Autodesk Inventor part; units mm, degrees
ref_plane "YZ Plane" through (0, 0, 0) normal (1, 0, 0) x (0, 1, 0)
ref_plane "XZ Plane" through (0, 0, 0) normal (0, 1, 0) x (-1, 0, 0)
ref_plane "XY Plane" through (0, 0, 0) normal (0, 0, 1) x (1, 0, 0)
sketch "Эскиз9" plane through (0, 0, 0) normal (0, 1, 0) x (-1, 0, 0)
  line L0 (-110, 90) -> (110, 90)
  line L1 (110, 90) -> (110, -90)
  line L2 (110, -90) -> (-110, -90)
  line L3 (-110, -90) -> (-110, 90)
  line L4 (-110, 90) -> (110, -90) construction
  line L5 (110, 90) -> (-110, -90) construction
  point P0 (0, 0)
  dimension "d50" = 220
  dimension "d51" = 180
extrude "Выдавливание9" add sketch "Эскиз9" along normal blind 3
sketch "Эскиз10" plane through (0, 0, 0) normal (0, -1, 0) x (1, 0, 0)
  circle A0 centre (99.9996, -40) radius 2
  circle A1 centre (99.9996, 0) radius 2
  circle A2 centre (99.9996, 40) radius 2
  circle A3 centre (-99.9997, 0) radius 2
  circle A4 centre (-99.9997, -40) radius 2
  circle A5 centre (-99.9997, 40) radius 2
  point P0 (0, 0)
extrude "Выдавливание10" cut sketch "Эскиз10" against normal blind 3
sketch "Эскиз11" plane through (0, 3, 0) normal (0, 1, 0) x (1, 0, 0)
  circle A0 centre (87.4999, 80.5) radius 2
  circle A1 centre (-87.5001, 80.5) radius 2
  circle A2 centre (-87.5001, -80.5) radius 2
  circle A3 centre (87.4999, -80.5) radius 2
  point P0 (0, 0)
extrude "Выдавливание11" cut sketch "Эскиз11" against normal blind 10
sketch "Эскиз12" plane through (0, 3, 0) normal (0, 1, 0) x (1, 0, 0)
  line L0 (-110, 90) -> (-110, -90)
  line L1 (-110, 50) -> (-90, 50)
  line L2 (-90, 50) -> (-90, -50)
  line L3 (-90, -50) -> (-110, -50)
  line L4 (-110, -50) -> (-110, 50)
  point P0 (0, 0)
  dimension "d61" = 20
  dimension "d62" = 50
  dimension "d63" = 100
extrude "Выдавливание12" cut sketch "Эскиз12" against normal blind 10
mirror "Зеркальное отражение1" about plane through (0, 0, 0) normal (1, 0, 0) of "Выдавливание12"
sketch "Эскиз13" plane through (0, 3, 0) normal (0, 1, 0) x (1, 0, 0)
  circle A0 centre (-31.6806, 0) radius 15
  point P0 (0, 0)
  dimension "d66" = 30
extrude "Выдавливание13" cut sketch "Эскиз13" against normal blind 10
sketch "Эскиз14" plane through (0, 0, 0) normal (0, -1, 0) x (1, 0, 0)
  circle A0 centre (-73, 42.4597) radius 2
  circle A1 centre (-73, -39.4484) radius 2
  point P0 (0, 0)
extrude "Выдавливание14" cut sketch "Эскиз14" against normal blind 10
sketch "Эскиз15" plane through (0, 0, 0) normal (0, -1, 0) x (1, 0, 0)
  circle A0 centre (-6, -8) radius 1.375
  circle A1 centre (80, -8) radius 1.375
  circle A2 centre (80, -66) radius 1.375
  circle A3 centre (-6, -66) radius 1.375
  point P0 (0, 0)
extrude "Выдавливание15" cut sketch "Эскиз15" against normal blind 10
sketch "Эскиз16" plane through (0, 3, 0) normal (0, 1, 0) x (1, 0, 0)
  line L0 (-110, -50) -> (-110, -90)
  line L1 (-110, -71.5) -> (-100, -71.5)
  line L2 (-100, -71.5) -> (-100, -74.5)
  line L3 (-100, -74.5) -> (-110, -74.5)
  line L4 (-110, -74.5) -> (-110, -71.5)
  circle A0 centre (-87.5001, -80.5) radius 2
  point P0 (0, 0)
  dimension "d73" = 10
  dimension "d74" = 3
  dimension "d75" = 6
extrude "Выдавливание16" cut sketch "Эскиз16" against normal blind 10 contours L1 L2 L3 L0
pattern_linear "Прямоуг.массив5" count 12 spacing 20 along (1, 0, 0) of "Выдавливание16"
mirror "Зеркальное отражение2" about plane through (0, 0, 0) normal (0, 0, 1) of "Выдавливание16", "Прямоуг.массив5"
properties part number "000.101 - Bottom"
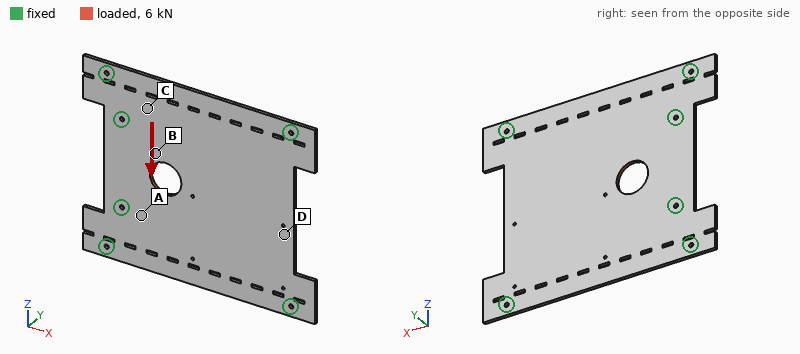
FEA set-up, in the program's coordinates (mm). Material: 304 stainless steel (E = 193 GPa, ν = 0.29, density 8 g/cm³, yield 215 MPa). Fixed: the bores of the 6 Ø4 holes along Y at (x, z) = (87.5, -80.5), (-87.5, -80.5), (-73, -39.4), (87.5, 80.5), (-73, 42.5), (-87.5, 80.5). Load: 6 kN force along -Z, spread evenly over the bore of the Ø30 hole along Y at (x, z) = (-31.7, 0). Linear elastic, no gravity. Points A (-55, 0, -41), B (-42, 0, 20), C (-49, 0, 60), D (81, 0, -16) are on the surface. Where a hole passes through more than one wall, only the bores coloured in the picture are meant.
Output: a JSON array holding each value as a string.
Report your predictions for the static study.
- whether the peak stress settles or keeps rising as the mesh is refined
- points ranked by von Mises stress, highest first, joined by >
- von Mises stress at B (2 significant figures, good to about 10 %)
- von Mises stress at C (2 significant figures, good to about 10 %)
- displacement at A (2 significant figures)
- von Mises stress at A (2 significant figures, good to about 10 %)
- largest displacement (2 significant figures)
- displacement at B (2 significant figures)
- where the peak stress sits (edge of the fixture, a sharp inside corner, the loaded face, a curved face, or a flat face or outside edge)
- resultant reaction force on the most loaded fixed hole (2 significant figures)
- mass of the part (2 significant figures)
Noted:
["keeps rising", "B > A > C > D", "21 MPa", "12 MPa", "3.8 µm", "16 MPa", "9.7 µm", "6.5 µm", "edge of the fixture", "1.9 kN", "820 g"]
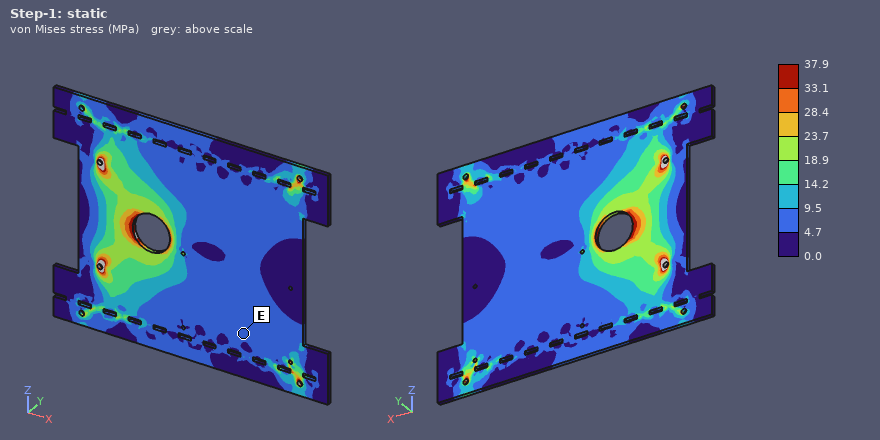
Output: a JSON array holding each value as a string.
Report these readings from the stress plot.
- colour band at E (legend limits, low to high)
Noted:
["4.7 to 9.5 MPa"]
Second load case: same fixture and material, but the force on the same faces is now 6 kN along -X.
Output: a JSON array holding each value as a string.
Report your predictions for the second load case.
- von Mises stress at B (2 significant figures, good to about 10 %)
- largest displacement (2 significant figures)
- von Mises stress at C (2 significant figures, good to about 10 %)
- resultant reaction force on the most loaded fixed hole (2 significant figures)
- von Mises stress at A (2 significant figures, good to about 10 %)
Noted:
["19 MPa", "7.8 µm", "6.2 MPa", "2.0 kN", "16 MPa"]
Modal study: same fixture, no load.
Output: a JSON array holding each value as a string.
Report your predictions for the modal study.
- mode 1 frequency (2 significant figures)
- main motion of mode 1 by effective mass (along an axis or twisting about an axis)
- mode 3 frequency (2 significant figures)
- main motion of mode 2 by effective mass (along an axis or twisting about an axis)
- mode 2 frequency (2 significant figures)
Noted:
["410 Hz", "along Y", "670 Hz", "twisting about X", "590 Hz"]
